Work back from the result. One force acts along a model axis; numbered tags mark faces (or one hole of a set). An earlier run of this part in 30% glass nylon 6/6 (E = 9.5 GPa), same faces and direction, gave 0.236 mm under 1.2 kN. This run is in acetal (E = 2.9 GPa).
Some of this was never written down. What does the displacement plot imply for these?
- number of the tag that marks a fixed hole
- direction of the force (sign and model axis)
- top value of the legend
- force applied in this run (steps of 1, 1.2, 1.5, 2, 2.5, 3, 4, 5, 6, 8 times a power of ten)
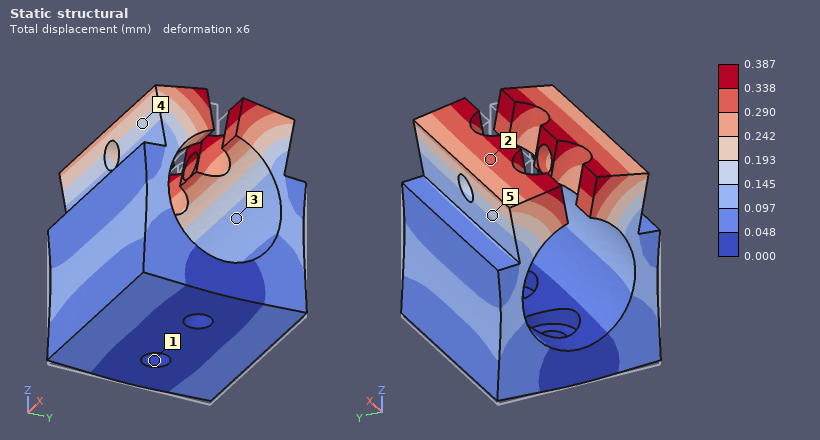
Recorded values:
1
+Z
0.387 mm
600 N
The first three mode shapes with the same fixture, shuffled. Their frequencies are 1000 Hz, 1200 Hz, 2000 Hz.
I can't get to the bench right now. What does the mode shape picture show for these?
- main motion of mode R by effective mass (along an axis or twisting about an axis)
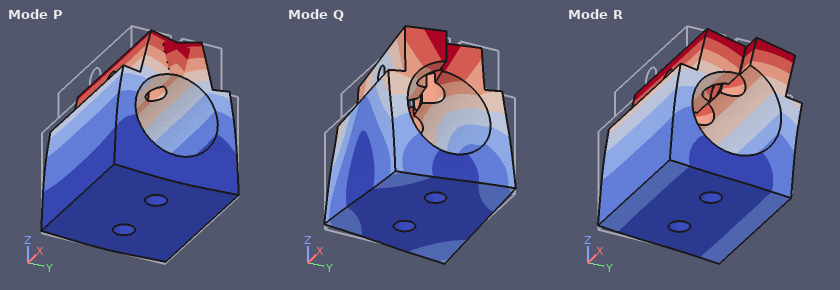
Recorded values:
along Y
